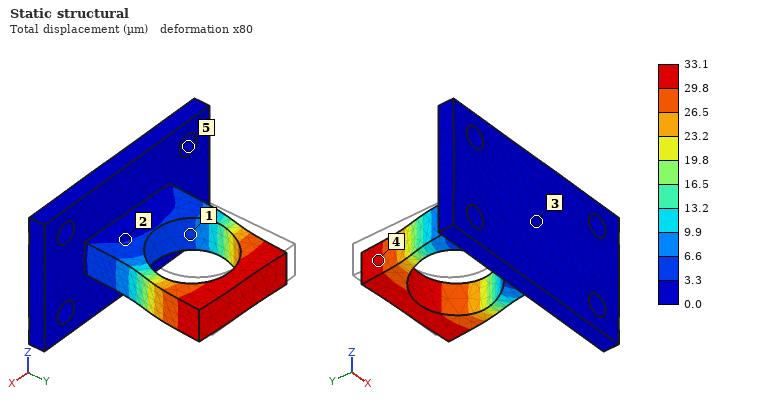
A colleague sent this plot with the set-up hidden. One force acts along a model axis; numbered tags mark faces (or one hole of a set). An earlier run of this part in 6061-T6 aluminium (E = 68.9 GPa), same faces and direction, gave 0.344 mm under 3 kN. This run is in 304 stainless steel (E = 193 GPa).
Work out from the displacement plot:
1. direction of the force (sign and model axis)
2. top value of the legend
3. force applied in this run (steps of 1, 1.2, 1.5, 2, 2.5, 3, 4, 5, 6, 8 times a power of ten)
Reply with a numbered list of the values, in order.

1. +X
2. 33.1 µm
3. 800 N
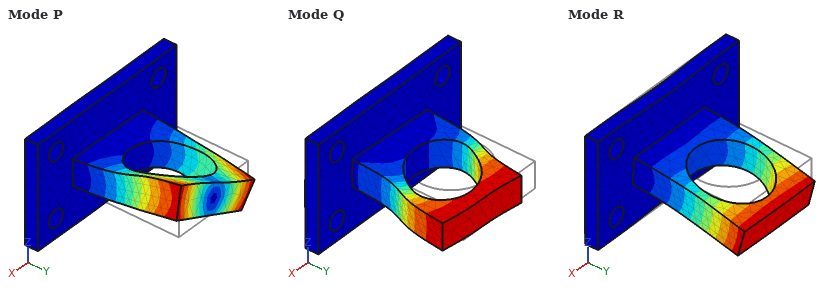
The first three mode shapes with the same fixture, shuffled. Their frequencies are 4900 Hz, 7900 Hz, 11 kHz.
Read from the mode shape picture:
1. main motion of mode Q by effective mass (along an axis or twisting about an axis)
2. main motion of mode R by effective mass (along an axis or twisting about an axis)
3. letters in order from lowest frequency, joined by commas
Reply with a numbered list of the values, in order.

1. along X
2. along Z
3. R, Q, P
